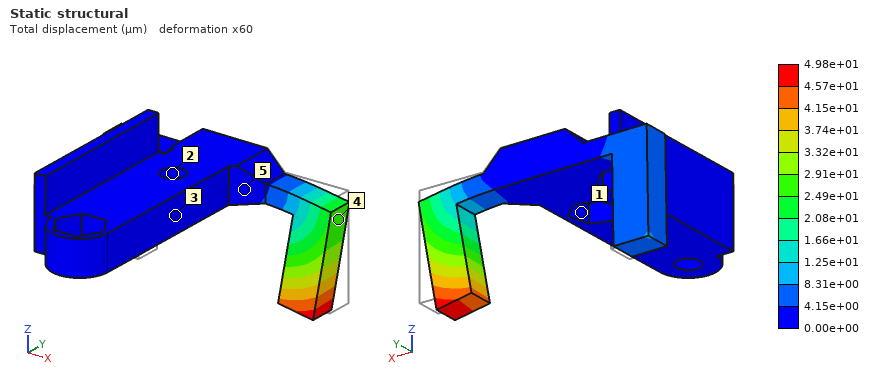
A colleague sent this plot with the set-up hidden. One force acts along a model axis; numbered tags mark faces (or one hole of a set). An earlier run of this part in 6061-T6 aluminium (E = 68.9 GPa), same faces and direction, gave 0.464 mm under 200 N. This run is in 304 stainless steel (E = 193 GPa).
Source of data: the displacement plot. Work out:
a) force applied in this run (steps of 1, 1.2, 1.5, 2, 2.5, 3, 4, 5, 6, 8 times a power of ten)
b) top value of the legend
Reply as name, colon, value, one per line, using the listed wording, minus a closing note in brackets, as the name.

force applied in this run: 60 N
top value of the legend: 4.98e+01 µm
